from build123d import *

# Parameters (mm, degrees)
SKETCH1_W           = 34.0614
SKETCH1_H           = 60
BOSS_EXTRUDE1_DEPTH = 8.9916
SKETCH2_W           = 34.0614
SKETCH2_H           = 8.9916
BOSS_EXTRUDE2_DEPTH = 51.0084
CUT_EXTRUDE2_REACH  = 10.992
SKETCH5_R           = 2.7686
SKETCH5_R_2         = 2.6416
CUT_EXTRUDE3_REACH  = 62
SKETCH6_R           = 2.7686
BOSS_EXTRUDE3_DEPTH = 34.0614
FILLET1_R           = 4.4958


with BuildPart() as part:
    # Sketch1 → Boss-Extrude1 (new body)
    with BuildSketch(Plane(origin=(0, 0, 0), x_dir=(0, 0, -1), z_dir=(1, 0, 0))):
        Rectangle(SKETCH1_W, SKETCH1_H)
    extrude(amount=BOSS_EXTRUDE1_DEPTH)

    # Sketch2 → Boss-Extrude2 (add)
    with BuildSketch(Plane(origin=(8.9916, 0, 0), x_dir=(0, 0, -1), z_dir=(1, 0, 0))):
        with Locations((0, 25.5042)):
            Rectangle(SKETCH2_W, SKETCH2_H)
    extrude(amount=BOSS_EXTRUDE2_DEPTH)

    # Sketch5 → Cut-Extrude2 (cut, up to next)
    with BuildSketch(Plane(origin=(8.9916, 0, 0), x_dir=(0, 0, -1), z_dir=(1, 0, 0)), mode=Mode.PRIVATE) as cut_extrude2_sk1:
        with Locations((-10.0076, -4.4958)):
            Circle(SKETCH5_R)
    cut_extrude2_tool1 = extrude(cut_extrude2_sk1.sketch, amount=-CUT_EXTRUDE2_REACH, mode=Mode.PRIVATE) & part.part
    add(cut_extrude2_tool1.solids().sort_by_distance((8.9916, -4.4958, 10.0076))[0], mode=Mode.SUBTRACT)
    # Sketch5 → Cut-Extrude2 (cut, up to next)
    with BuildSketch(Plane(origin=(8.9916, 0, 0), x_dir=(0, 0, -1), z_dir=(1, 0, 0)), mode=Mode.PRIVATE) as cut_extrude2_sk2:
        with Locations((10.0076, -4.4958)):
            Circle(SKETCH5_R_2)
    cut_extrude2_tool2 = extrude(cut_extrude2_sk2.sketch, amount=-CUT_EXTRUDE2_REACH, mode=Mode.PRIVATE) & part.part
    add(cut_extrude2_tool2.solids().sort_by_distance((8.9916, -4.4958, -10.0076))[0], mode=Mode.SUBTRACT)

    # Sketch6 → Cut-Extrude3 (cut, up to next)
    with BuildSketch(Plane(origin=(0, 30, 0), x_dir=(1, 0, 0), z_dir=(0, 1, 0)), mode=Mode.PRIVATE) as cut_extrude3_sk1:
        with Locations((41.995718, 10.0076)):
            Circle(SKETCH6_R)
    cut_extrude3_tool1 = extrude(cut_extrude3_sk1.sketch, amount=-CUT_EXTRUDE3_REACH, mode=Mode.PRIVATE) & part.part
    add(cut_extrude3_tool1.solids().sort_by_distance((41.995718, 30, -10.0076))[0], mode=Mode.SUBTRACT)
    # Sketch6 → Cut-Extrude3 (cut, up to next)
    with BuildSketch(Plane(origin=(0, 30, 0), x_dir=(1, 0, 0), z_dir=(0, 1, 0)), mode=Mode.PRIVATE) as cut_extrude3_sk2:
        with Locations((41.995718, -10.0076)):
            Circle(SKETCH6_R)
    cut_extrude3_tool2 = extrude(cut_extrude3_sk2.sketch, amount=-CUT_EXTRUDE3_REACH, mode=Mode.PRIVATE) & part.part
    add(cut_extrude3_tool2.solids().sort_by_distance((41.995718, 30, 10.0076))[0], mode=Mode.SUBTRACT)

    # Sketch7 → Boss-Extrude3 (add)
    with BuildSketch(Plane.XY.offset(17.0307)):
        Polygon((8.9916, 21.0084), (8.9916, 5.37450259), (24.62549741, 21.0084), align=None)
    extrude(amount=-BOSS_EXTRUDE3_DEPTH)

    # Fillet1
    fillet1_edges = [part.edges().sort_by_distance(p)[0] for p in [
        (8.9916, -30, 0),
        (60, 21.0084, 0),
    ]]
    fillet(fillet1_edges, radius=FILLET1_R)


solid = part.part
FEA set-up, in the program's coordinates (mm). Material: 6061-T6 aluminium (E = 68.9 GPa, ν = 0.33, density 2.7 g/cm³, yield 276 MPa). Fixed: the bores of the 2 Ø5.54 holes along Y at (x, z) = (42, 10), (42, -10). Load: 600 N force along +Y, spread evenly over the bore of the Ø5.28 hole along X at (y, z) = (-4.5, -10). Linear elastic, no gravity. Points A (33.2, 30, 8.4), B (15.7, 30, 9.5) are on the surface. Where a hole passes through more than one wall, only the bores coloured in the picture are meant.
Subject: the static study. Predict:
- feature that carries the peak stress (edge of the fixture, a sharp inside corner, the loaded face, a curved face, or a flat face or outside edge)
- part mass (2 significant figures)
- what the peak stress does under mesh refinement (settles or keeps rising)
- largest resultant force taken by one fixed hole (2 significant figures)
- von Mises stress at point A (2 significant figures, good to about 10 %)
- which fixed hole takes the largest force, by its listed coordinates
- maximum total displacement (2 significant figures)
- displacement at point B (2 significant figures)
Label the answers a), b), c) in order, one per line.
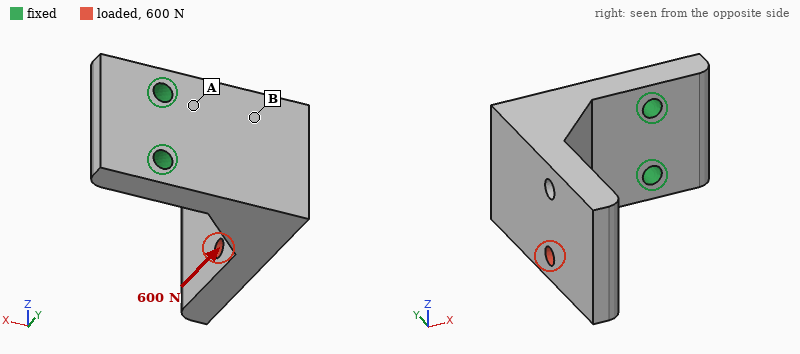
a) edge of the fixture
b) 100 g
c) keeps rising
d) 530 N
e) 36 MPa
f) (42, -10)
g) 0.16 mm
h) 0.038 mm
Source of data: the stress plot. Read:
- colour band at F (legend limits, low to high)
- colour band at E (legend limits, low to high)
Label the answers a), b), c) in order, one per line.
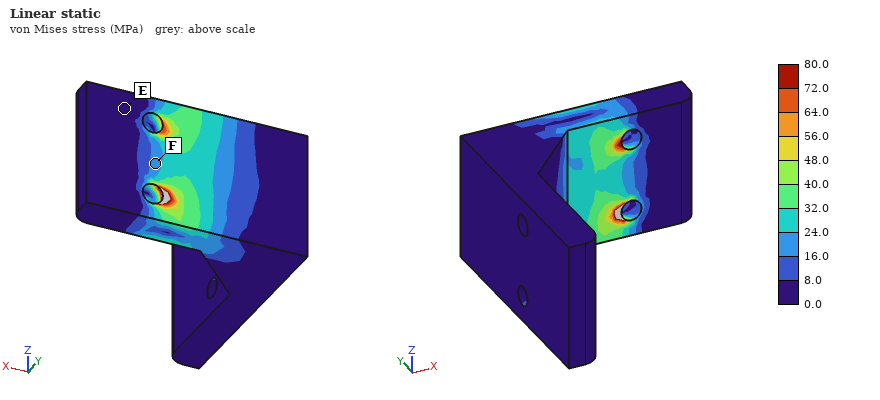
a) 16.0 to 24.0 MPa
b) 0.0 to 8.0 MPa
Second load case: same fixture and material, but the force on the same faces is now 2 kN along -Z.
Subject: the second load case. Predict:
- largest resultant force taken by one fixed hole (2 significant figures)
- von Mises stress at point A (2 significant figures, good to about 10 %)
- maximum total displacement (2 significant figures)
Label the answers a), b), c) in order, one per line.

a) 4.1 kN
b) 60 MPa
c) 0.26 mm
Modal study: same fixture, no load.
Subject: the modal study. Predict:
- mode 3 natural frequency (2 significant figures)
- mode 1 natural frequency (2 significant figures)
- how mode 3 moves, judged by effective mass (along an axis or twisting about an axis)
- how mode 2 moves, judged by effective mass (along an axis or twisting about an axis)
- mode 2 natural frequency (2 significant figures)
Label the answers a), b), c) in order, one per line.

a) 4900 Hz
b) 1400 Hz
c) along Y
d) along Z
e) 2500 Hz
